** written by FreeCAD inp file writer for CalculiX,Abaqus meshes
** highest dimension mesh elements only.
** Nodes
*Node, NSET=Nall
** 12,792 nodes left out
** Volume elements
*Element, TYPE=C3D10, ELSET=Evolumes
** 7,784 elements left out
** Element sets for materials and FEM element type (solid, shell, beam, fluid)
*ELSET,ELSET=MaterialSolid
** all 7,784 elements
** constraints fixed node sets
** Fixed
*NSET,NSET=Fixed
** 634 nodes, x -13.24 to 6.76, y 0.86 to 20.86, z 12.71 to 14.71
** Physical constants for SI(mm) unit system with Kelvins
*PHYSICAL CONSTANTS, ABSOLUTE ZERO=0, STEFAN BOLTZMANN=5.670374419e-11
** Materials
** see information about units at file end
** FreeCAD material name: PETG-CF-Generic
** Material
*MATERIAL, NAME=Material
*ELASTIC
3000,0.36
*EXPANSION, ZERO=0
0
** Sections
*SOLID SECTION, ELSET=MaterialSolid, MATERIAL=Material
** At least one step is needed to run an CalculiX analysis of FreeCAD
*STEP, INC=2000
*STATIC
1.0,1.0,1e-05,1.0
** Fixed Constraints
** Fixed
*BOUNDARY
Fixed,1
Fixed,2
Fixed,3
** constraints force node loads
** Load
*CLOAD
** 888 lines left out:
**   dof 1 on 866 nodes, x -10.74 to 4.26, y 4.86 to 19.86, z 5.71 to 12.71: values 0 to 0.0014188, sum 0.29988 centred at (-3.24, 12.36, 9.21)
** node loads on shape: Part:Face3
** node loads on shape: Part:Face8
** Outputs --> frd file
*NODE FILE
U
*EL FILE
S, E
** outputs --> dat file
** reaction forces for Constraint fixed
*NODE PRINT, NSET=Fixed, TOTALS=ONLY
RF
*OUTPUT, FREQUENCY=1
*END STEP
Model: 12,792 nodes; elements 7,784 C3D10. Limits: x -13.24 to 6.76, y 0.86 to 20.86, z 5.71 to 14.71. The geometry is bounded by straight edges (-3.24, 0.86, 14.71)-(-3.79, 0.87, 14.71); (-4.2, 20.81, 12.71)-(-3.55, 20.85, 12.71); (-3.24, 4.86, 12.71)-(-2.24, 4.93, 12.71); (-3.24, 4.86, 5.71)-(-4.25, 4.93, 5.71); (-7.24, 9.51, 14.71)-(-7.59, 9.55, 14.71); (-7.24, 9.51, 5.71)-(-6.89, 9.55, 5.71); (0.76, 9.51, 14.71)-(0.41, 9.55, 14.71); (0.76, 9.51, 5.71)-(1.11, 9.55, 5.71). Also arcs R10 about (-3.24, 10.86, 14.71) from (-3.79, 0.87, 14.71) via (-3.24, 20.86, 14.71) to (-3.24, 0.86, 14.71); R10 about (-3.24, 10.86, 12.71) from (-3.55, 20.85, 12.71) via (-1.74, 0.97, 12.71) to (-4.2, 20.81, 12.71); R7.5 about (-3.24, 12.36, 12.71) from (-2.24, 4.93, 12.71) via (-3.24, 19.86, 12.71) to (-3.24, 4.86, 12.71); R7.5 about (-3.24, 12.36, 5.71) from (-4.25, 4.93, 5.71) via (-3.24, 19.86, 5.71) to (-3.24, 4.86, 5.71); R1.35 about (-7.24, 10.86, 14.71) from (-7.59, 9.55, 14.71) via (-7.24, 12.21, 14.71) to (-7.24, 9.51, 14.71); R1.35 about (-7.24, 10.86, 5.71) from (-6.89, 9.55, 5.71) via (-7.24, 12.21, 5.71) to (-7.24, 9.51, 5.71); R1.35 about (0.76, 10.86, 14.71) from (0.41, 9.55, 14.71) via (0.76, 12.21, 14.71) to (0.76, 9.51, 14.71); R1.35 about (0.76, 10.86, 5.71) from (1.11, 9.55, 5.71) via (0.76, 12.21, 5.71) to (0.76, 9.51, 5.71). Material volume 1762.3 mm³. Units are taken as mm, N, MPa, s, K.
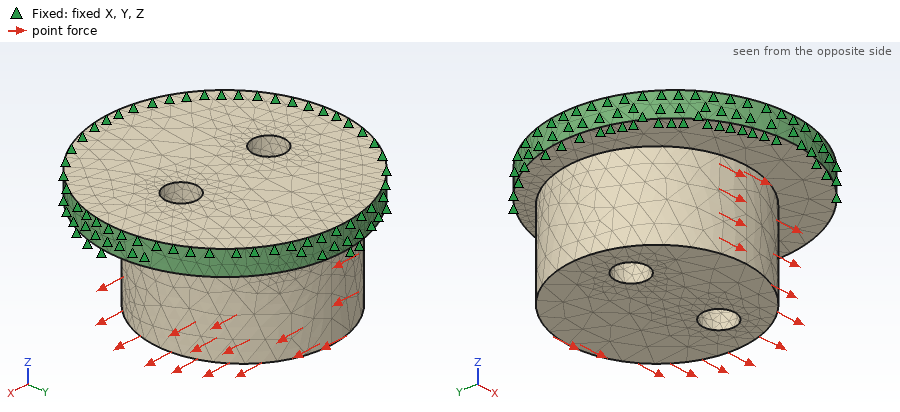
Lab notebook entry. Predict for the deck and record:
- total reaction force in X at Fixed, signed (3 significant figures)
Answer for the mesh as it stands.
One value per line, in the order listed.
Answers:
-0.300 N
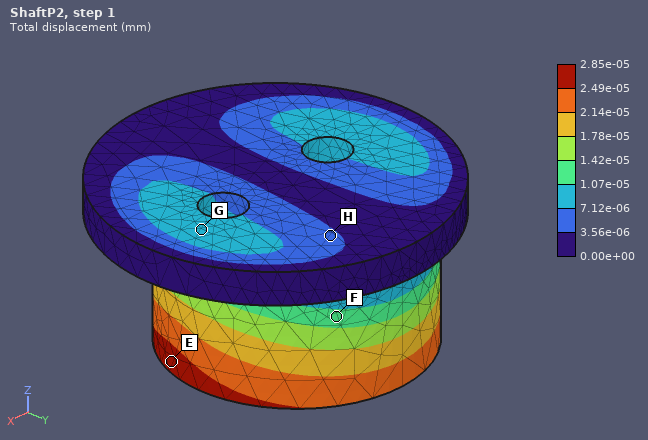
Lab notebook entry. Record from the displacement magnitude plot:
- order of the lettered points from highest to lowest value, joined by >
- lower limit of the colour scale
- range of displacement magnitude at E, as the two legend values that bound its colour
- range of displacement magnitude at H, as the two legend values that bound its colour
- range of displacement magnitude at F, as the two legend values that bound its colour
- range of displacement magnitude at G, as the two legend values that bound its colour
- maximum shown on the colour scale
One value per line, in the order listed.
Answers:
E > F > G > H
0.00e+00 mm
2.49e-05 to 2.85e-05 mm
3.56e-06 to 7.12e-06 mm
1.07e-05 to 1.42e-05 mm
7.12e-06 to 1.07e-05 mm
2.85e-05 mm
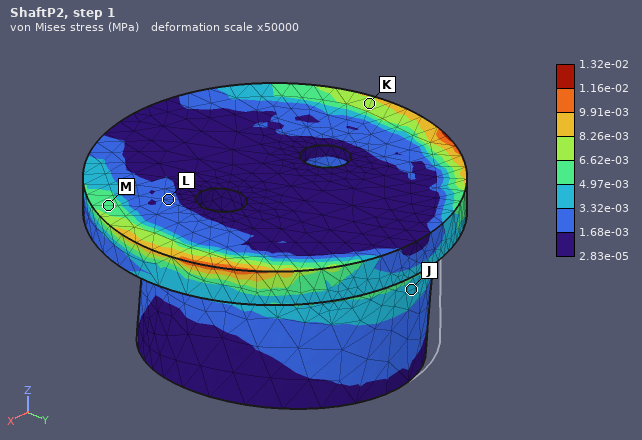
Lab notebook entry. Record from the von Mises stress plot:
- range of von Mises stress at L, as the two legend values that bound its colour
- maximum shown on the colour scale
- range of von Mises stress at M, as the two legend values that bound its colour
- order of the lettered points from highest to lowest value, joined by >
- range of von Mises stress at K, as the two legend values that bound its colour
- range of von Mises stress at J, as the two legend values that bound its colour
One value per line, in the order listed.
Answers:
1.68e-03 to 3.32e-03 MPa
1.32e-02 MPa
4.97e-03 to 6.62e-03 MPa
K > M > J > L
6.62e-03 to 8.26e-03 MPa
3.32e-03 to 4.97e-03 MPa
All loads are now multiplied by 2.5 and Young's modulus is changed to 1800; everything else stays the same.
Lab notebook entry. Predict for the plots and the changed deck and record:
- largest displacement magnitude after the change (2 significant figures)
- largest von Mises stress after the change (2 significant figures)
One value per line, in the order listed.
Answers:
1.2e-04 mm
0.033 MPa
